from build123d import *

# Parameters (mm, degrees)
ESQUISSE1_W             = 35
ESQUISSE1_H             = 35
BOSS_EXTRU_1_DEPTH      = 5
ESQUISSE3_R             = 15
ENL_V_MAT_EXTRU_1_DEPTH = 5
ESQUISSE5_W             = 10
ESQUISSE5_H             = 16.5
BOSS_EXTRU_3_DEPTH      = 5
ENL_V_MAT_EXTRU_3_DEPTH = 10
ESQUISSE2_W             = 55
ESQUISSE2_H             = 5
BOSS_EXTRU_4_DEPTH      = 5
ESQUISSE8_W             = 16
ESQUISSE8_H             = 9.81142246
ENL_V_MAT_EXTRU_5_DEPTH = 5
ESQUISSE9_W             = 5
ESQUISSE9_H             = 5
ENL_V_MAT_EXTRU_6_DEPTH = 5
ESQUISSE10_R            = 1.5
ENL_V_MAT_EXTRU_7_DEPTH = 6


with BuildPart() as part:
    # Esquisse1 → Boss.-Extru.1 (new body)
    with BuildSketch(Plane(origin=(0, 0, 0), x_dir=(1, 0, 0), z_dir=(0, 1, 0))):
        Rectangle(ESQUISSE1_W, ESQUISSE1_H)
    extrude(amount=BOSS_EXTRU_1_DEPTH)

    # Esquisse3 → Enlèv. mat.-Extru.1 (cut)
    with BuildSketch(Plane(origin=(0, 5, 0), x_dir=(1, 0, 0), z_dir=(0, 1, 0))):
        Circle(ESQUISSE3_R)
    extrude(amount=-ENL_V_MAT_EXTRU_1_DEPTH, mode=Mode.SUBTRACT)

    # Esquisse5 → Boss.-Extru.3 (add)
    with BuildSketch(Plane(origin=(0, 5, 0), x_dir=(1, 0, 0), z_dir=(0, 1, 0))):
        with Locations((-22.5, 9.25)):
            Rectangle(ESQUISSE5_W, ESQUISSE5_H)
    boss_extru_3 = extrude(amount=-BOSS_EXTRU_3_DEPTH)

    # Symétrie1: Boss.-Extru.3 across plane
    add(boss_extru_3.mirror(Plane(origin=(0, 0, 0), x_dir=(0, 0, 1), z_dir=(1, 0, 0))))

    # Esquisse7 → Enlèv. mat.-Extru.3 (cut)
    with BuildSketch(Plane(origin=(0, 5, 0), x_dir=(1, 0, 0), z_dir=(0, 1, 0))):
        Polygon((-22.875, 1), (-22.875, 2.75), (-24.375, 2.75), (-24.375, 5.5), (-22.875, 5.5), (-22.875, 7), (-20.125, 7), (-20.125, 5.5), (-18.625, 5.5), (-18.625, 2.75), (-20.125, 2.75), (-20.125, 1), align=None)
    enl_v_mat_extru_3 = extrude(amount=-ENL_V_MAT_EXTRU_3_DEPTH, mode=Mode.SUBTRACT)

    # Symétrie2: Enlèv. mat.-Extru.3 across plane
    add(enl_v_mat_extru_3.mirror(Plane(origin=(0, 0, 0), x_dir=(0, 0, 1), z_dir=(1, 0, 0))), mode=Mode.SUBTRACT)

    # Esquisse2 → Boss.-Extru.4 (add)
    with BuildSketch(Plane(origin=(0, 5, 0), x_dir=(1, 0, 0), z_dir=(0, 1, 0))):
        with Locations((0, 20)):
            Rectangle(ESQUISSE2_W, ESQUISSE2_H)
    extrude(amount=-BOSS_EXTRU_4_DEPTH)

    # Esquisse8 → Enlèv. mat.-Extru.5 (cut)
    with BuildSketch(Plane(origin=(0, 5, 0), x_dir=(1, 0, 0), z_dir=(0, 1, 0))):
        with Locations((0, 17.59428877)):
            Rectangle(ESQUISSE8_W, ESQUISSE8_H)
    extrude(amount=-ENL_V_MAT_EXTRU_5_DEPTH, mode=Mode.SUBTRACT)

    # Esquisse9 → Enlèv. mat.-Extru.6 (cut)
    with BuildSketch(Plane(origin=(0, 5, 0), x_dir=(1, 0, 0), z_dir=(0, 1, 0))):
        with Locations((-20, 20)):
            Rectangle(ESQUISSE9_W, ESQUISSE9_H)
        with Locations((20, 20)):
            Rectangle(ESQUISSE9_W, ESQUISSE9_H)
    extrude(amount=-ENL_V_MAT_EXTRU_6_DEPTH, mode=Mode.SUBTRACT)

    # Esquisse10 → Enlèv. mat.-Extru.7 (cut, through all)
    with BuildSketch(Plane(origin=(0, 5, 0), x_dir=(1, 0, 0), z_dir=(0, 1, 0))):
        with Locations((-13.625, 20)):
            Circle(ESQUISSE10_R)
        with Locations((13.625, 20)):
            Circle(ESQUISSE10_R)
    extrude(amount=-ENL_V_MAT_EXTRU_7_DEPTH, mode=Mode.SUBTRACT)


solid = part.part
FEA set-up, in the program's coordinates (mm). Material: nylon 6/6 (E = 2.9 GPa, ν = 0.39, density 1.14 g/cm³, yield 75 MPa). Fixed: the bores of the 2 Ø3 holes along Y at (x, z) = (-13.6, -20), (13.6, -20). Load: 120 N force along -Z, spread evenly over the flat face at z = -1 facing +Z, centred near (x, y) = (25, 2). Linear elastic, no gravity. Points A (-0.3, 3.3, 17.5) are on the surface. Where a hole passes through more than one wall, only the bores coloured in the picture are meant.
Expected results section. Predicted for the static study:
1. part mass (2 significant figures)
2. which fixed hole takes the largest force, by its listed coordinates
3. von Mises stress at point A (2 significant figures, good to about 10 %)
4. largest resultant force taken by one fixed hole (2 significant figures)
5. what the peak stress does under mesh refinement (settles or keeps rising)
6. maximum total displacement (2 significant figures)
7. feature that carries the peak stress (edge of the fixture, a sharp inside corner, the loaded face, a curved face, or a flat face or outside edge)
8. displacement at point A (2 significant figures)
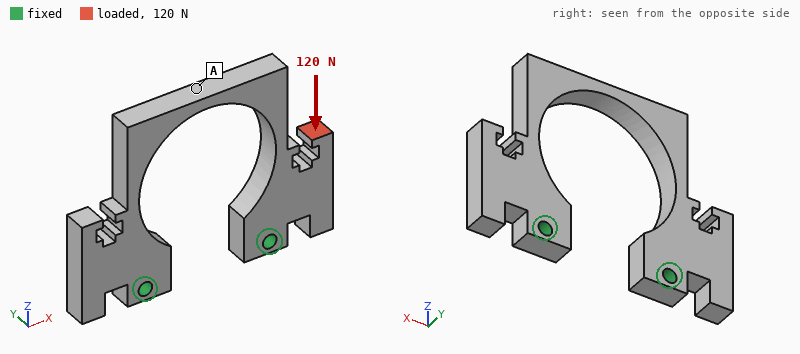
5.0 g
(13.6, -20)
5.5 MPa
120 N
keeps rising
0.41 mm
edge of the fixture
0.25 mm
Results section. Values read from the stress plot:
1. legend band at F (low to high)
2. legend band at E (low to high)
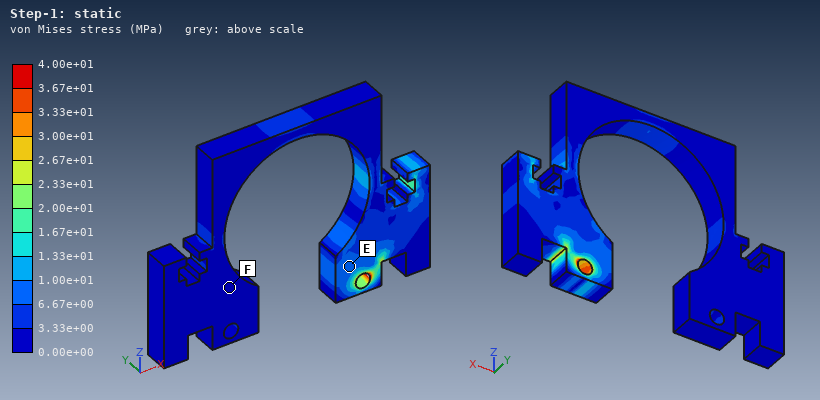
0.00e+00 to 3.33e+00 MPa
6.67e+00 to 1.00e+01 MPa
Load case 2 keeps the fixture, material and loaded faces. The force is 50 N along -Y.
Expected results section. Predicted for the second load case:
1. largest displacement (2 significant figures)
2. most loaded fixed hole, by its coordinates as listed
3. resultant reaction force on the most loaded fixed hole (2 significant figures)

0.79 mm
(13.6, -20)
49 N
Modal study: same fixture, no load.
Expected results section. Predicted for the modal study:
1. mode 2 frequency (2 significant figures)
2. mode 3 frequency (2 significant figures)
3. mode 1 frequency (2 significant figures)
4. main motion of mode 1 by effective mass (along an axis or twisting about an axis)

1400 Hz
1400 Hz
750 Hz
along Y
